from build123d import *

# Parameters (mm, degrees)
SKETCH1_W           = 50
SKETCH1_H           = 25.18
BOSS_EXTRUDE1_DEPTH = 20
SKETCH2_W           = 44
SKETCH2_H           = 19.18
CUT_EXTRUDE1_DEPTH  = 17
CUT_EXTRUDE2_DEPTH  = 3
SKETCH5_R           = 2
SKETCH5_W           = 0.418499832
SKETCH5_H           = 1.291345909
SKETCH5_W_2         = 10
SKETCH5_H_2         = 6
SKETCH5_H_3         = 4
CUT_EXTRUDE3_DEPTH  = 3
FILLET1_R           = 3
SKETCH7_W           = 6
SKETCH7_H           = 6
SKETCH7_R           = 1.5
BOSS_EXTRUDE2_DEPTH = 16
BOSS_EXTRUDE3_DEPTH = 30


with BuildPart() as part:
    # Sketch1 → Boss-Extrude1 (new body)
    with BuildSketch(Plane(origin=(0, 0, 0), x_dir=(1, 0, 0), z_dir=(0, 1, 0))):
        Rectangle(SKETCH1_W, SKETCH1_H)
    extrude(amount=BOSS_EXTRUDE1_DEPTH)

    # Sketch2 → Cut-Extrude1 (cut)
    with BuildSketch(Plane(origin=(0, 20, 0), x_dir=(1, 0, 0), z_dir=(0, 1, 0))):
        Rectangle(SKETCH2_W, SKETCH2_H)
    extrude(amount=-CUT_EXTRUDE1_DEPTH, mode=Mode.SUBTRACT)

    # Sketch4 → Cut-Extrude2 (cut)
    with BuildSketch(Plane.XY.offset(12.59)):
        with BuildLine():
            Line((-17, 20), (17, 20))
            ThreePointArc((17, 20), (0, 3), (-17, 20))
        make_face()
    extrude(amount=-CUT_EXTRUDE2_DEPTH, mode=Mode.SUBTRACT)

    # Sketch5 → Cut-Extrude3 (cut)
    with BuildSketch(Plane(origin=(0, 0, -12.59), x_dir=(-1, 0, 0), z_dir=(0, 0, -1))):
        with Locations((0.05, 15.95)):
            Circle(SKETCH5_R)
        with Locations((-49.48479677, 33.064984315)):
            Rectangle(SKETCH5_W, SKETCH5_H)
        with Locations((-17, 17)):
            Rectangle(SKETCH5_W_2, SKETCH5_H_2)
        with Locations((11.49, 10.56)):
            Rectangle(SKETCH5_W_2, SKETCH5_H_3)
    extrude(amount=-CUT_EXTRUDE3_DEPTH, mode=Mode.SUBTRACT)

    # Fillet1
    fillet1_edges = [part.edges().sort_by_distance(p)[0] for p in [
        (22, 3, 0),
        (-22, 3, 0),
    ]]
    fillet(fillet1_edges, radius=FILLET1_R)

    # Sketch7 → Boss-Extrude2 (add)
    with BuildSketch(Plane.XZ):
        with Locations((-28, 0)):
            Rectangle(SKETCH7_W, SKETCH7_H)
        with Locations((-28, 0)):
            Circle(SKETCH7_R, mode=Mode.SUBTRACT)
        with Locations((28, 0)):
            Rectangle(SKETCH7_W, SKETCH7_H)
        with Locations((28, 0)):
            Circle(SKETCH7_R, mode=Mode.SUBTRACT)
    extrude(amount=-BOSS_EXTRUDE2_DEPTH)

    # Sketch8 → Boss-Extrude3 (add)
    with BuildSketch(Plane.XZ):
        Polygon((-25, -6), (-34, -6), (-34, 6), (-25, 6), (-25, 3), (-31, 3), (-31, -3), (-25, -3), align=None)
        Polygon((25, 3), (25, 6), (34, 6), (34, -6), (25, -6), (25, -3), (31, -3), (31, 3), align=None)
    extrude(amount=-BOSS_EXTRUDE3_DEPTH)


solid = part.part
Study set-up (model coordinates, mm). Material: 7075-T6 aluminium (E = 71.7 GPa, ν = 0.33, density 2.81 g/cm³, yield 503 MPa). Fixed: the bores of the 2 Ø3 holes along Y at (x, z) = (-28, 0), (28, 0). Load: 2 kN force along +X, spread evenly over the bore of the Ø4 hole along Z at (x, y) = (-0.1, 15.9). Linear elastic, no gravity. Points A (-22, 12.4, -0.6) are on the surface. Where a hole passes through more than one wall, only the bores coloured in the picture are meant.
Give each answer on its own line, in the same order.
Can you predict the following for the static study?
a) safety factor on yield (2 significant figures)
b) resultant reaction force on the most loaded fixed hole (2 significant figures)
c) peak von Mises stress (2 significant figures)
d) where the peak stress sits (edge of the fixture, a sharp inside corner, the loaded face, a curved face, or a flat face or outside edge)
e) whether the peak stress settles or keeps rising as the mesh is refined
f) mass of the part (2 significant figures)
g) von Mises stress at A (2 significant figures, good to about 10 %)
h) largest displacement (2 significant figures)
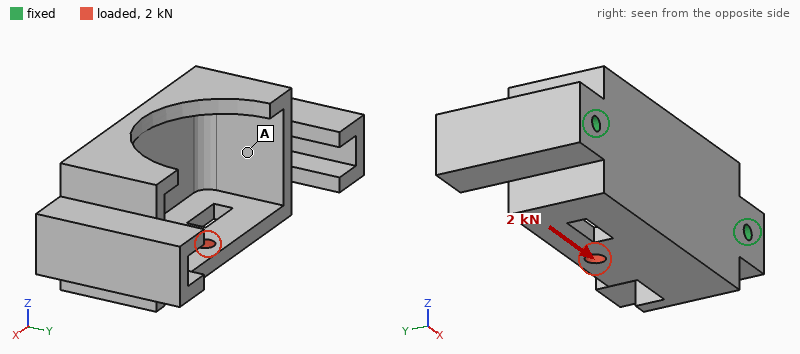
5.2
1.2 kN
98 MPa
the loaded face
settles
41 g
14 MPa
28 µm
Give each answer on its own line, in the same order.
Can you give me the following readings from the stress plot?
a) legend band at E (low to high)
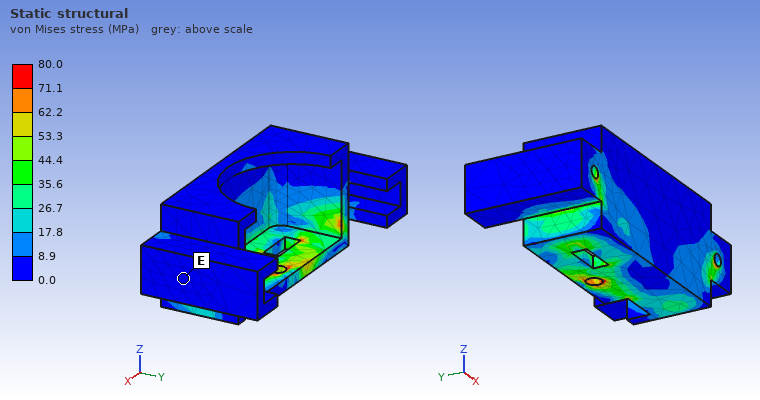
0.0 to 8.9 MPa
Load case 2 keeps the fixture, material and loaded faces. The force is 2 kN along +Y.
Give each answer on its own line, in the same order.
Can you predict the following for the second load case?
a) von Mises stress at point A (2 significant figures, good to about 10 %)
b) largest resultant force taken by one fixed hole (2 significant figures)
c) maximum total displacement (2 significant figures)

11 MPa
1.0 kN
60 µm
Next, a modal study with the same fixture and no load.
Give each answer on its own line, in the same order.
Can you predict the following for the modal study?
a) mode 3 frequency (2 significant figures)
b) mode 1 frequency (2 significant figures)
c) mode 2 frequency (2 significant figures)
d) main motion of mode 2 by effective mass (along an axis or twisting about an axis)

15 kHz
8700 Hz
12 kHz
along Y
